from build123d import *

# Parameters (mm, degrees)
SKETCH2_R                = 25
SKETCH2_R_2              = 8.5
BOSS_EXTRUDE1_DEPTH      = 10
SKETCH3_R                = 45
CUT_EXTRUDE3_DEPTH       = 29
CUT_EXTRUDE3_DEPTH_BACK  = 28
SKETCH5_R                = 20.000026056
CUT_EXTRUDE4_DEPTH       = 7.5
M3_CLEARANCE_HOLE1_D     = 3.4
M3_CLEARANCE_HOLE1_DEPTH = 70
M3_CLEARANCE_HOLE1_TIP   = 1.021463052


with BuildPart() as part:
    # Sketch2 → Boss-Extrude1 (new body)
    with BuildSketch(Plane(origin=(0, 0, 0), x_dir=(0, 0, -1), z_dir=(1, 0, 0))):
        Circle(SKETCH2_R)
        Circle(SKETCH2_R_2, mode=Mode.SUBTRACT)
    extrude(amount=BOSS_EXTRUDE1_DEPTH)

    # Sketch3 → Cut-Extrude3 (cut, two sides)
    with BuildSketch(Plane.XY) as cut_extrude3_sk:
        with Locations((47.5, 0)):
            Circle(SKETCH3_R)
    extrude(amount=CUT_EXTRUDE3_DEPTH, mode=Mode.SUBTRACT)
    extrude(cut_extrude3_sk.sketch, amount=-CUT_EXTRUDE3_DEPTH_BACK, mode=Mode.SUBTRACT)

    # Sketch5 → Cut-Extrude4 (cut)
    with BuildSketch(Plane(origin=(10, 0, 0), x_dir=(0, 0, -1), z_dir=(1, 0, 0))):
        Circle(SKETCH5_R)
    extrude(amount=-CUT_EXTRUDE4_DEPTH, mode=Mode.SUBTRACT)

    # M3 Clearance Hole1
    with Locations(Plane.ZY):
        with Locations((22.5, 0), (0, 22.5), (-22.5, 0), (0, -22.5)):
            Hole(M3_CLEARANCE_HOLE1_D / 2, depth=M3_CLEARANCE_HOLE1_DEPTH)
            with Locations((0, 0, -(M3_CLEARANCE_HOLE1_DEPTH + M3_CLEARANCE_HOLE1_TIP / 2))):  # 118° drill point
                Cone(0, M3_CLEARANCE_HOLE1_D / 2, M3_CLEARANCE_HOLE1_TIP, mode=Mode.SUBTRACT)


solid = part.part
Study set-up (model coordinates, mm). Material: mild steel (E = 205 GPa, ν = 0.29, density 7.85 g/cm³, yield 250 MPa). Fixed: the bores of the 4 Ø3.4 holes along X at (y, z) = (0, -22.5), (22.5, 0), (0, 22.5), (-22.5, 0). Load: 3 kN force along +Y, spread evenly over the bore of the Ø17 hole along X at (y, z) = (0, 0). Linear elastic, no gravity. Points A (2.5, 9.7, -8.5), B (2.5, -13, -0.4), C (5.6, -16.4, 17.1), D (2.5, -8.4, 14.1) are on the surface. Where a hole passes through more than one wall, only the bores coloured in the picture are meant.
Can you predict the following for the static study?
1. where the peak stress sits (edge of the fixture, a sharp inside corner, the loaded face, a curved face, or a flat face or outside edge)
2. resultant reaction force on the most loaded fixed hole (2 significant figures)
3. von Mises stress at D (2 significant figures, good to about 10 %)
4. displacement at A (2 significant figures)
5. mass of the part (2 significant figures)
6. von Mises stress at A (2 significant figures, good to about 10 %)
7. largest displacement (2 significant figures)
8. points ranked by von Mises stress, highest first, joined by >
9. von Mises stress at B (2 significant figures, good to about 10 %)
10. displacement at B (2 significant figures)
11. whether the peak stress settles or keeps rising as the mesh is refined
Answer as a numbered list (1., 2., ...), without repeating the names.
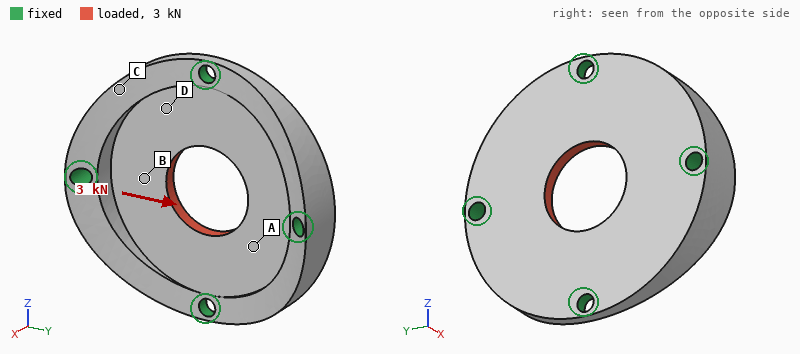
1. edge of the fixture
2. 920 N
3. 12 MPa
4. 2.0 µm
5. 49 g
6. 23 MPa
7. 2.8 µm
8. B > A > D > C
9. 33 MPa
10. 1.5 µm
11. keeps rising
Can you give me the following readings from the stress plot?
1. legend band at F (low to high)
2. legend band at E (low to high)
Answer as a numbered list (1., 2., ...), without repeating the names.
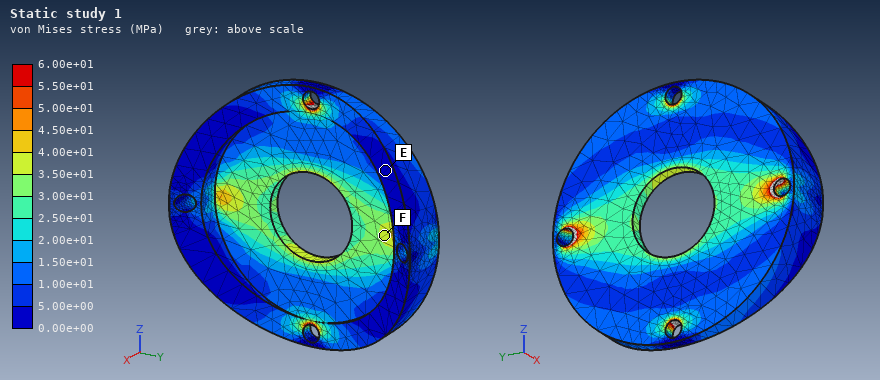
1. 3.50e+01 to 4.00e+01 MPa
2. 0.00e+00 to 5.00e+00 MPa
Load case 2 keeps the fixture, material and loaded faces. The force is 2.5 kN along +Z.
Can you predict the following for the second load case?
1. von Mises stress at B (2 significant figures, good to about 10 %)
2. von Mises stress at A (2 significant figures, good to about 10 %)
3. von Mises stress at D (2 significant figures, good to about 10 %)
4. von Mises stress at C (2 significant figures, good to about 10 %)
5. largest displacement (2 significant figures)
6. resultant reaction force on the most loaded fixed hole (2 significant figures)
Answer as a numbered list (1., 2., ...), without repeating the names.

1. 11 MPa
2. 16 MPa
3. 14 MPa
4. 5.4 MPa
5. 2.2 µm
6. 680 N
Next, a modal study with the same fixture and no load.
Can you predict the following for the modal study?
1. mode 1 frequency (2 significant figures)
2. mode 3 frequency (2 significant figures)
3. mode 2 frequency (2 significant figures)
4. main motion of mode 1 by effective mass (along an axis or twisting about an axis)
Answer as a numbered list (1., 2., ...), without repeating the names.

1. 14 kHz
2. 19 kHz
3. 18 kHz
4. along X
